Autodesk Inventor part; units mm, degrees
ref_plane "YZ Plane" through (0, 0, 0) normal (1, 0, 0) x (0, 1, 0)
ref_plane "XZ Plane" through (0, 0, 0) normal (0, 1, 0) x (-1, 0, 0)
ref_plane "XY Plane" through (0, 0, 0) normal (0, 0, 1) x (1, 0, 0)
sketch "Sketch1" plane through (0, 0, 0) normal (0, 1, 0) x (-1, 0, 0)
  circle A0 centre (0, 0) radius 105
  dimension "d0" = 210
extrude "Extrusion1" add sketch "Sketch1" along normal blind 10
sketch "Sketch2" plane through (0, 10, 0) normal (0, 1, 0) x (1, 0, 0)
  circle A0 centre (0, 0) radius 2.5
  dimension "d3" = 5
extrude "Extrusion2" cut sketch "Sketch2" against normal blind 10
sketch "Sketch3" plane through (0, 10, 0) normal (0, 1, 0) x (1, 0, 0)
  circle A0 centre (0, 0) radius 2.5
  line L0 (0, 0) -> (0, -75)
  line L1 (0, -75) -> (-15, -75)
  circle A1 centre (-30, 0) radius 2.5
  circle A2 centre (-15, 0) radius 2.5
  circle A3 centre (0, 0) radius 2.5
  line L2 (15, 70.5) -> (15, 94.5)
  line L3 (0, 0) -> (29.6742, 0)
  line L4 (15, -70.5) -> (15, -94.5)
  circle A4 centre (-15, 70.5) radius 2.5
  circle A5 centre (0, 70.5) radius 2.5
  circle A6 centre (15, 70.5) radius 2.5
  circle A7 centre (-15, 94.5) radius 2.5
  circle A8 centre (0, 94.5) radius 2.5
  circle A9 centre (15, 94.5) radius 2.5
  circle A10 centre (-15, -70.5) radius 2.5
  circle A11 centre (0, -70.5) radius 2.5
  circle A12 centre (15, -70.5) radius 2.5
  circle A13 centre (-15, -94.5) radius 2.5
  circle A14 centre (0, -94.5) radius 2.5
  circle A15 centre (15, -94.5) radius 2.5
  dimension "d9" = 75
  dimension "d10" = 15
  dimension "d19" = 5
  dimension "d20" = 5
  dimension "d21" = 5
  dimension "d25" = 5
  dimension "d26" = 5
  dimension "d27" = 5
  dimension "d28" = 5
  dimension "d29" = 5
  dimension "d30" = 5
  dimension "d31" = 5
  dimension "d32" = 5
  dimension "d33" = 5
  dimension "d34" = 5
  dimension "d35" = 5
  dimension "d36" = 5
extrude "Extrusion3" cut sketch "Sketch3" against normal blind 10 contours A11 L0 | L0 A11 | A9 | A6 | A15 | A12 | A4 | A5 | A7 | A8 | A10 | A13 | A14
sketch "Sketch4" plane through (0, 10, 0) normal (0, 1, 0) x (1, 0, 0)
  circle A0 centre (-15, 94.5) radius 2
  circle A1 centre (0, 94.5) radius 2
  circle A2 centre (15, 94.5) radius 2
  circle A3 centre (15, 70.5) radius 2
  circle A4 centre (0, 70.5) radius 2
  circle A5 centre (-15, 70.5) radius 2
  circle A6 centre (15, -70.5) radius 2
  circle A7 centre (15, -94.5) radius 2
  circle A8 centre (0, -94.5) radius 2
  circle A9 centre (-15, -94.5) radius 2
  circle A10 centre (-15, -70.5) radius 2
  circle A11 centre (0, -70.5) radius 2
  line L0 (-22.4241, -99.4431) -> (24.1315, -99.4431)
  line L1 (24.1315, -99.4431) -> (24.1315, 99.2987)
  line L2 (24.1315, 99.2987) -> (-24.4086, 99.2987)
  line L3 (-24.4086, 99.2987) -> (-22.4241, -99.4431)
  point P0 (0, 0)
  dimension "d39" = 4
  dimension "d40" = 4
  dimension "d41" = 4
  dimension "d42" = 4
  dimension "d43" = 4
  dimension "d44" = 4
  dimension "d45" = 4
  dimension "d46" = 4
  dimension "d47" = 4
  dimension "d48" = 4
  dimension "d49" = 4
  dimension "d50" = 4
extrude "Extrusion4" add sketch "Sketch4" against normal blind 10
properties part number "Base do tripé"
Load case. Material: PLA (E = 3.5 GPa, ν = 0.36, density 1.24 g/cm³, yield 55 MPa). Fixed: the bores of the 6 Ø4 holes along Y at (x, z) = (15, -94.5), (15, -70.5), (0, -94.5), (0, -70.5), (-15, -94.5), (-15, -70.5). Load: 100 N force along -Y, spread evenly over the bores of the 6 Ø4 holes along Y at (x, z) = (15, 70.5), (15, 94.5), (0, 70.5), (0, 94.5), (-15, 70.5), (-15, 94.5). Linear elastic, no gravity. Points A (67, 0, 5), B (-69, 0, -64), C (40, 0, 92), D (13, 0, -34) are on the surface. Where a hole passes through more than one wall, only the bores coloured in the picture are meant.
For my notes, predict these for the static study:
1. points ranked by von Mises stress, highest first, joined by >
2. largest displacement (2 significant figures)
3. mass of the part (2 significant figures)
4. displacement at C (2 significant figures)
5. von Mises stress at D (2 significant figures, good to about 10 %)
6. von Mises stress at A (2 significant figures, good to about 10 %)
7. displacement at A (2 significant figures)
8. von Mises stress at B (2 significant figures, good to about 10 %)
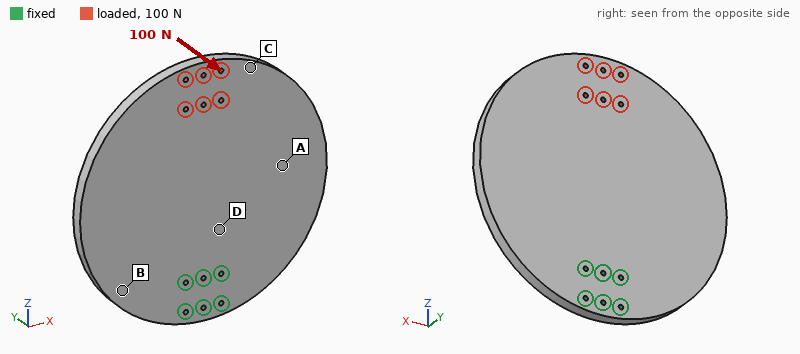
D > B > A > C
3.5 mm
430 g
3.0 mm
4.0 MPa
2.1 MPa
0.96 mm
3.3 MPa
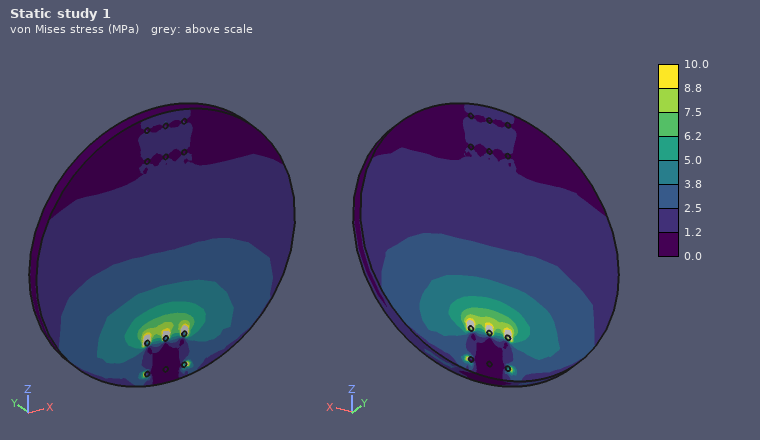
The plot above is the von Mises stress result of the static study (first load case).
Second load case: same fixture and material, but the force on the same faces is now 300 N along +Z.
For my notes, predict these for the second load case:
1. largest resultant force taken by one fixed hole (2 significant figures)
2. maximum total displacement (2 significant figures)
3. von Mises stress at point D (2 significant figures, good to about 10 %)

89 N
17 µm
0.35 MPa
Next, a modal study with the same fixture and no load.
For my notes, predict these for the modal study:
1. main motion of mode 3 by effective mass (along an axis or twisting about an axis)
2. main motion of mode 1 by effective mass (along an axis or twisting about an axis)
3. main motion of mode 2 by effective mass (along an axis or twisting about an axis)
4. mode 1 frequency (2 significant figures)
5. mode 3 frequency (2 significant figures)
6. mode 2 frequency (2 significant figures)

along Y
along Y
twisting about Z
89 Hz
360 Hz
160 Hz
